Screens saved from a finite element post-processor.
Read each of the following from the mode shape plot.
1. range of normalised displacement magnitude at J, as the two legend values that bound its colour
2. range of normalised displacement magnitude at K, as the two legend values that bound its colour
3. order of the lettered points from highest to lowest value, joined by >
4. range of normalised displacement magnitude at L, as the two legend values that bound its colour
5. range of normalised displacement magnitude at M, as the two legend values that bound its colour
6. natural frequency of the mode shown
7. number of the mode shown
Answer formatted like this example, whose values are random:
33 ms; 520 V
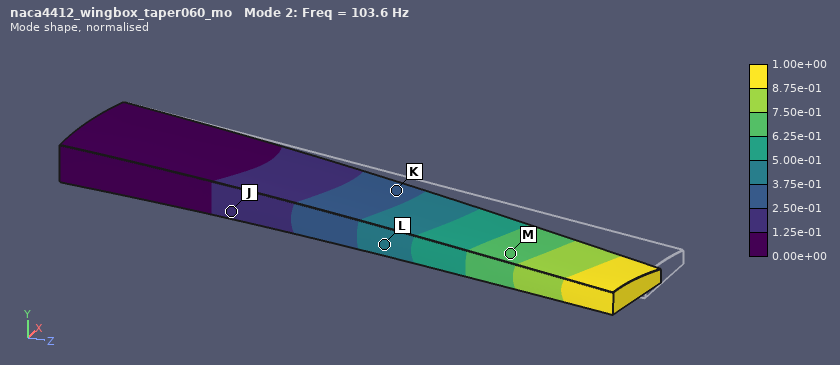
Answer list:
1.25e-01 to 2.50e-01; 2.50e-01 to 3.75e-01; M > L > K > J; 3.75e-01 to 5.00e-01; 6.25e-01 to 7.50e-01; 103.6 Hz; 2
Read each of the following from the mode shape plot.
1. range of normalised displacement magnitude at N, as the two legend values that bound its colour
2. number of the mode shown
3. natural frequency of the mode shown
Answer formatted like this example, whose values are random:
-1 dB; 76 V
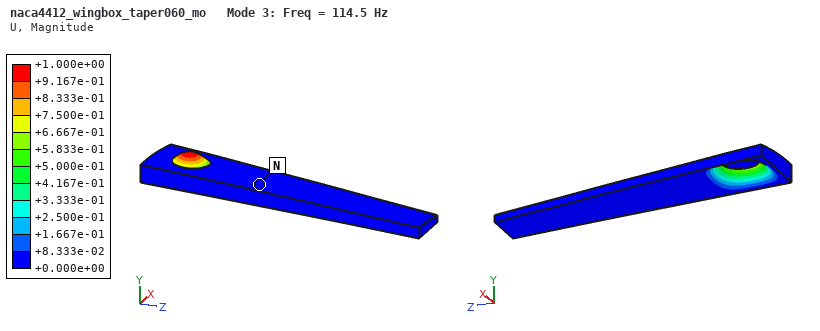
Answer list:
+0.000e+00 to +8.333e-02; 3; 114.5 Hz
